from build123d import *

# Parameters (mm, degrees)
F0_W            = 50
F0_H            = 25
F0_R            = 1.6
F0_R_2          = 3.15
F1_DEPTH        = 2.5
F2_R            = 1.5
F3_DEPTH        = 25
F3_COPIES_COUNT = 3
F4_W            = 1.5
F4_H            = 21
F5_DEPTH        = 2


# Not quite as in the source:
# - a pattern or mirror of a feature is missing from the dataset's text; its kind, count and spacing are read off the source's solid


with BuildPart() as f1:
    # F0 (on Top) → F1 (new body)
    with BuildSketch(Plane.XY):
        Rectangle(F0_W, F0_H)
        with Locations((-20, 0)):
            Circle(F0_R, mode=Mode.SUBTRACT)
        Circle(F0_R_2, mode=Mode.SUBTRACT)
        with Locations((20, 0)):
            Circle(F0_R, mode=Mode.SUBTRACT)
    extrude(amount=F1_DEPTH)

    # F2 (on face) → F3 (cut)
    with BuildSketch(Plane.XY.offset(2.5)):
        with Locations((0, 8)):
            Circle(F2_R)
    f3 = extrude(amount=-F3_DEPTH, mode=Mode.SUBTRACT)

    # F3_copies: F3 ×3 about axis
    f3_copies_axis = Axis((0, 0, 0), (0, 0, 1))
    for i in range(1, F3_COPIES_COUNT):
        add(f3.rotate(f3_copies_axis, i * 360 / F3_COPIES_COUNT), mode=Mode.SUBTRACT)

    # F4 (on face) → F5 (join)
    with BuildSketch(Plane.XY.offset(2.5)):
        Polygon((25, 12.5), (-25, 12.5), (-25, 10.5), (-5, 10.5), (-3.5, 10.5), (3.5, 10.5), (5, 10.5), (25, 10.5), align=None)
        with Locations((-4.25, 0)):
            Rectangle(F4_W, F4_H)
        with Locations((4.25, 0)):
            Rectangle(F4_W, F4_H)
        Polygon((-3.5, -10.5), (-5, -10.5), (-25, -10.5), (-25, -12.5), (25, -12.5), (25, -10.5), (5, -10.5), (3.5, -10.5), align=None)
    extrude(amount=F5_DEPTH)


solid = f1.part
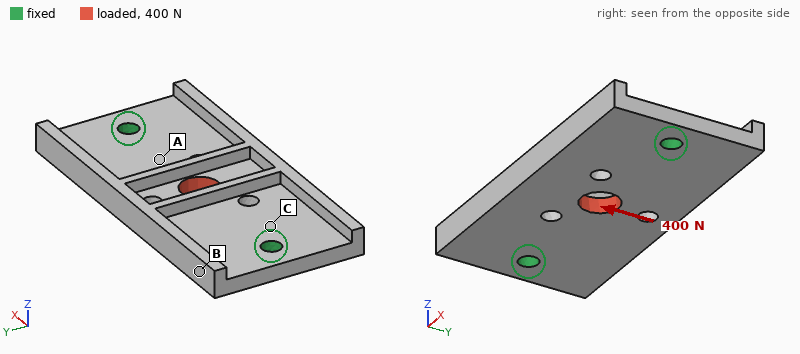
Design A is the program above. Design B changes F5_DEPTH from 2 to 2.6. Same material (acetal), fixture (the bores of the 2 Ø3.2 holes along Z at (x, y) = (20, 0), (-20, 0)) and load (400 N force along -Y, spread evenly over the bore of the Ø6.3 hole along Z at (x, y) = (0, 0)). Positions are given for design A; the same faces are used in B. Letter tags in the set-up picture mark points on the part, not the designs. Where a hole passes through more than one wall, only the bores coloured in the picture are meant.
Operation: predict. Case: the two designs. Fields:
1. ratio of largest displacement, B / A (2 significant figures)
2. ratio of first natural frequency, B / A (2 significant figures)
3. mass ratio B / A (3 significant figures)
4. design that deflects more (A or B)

1.1
0.98
1.05
B
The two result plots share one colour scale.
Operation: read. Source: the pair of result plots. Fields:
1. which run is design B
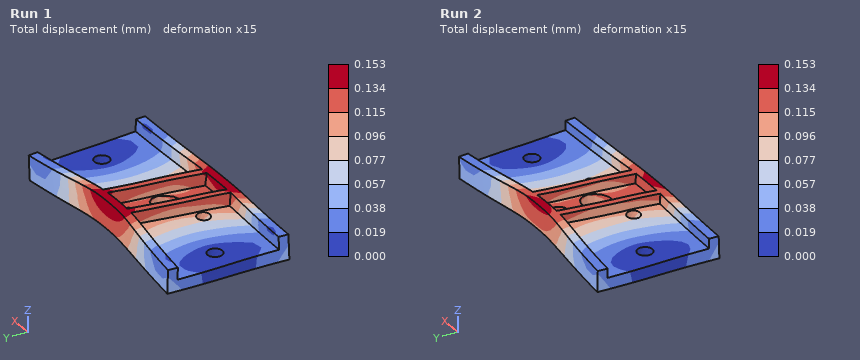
Run 1
